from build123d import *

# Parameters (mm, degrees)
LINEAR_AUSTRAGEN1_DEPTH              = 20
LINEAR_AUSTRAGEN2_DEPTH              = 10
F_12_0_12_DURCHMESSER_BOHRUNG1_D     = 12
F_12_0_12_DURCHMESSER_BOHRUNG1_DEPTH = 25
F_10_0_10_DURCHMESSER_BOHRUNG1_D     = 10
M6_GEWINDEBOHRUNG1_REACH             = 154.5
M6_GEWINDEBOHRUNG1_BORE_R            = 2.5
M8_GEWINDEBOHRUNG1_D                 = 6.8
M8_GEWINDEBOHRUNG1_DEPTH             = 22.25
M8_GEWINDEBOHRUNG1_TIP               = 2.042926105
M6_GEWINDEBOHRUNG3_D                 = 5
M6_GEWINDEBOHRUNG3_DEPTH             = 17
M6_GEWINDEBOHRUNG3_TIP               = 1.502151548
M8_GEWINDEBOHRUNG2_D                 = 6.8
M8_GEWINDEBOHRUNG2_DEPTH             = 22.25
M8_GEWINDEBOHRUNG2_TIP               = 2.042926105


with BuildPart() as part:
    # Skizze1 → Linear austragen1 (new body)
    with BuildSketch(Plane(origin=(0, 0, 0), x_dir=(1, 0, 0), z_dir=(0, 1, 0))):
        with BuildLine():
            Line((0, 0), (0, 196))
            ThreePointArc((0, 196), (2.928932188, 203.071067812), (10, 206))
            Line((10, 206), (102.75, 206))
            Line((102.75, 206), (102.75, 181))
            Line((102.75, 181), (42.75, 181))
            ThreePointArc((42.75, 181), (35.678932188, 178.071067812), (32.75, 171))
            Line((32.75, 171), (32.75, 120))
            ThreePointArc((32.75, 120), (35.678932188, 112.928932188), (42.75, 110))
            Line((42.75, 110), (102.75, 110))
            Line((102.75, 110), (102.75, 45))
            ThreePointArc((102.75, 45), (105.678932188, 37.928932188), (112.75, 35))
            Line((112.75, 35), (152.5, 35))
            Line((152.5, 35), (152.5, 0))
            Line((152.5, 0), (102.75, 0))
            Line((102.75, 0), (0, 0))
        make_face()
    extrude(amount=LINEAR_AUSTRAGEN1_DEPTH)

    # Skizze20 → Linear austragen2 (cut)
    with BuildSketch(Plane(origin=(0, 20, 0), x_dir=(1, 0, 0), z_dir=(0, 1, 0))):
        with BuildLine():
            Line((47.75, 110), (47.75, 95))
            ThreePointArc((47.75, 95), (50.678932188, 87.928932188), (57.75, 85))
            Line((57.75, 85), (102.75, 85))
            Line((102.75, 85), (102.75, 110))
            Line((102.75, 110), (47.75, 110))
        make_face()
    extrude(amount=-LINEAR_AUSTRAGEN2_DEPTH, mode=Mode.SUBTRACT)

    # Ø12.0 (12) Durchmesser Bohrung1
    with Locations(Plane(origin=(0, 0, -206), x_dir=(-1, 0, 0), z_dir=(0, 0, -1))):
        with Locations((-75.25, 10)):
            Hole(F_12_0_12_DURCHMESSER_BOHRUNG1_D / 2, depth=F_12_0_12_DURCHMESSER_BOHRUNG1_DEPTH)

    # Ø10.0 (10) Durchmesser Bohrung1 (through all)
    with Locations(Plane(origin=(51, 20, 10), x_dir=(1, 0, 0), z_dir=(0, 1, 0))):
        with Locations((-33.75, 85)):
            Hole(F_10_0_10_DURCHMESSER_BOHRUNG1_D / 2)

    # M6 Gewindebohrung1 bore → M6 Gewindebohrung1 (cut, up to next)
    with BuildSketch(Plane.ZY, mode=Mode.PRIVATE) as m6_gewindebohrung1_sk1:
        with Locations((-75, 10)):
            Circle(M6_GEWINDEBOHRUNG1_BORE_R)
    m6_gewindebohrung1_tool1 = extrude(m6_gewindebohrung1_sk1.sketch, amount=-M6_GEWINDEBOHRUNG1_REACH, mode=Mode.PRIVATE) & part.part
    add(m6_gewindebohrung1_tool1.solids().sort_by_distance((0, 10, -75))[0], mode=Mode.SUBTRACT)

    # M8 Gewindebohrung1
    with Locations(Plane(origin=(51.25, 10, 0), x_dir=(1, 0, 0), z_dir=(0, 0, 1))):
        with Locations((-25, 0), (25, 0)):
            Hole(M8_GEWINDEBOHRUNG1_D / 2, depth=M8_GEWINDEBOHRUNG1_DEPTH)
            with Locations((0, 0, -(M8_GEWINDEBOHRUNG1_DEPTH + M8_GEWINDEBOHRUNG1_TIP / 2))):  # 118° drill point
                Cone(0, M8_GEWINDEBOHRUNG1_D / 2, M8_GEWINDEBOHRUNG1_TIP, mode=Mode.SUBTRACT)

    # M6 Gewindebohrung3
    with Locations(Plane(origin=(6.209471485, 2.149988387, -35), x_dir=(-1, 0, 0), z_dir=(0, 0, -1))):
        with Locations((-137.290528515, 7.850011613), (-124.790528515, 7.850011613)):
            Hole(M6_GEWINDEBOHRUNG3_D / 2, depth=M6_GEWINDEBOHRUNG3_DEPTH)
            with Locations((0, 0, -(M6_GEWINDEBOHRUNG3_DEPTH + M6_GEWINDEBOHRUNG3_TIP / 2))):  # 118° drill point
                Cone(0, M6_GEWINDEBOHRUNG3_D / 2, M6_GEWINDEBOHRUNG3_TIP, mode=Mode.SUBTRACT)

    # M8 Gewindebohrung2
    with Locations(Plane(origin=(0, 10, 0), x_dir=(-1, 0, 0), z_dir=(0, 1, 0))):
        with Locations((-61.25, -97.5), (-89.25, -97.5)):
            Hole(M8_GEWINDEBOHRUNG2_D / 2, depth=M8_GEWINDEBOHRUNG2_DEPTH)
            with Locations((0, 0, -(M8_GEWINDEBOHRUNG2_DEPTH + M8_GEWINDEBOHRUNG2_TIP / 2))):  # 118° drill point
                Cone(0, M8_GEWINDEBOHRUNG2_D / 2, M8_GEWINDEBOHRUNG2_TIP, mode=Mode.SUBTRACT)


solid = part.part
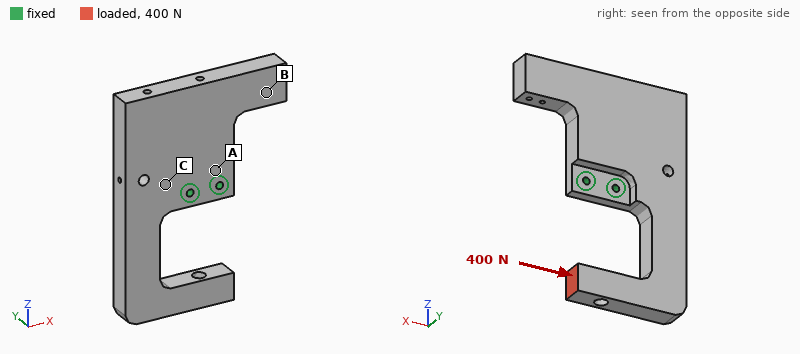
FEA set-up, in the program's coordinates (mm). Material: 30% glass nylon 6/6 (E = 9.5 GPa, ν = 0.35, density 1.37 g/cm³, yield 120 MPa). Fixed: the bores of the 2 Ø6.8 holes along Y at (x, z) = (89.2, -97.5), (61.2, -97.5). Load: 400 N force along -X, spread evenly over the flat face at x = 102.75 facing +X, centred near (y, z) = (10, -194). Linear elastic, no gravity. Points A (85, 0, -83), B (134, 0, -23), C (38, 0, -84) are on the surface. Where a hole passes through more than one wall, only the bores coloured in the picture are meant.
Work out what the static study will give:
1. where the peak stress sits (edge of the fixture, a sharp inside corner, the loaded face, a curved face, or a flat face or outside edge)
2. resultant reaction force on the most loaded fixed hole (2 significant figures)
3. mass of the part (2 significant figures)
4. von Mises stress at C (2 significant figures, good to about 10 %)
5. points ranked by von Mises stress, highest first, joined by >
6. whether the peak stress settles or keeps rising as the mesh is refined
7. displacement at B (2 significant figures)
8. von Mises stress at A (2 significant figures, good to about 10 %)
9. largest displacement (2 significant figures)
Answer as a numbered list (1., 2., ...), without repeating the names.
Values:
1. edge of the fixture
2. 1.3 kN
3. 460 g
4. 3.0 MPa
5. A > C > B
6. keeps rising
7. 0.11 mm
8. 4.6 MPa
9. 0.57 mm
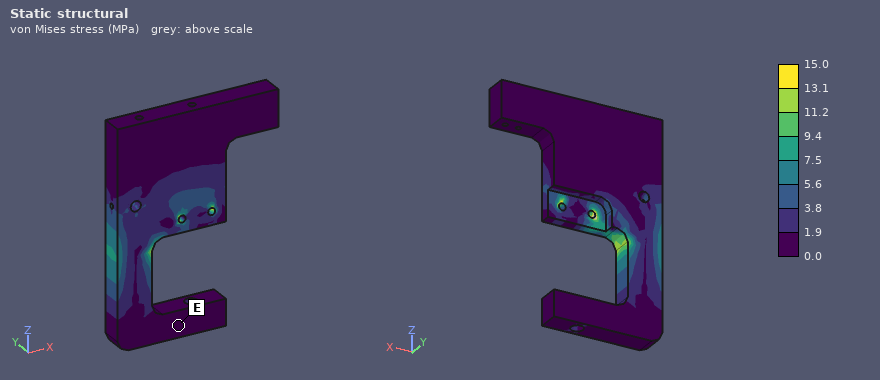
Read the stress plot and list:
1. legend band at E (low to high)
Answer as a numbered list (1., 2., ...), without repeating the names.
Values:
1. 0.0 to 1.9 MPa
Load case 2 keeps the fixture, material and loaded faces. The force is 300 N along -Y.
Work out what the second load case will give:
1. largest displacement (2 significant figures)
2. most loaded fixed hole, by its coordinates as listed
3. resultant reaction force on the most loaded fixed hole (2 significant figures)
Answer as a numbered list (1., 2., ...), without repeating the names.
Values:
1. 3.1 mm
2. (89.2, -97.5)
3. 360 N
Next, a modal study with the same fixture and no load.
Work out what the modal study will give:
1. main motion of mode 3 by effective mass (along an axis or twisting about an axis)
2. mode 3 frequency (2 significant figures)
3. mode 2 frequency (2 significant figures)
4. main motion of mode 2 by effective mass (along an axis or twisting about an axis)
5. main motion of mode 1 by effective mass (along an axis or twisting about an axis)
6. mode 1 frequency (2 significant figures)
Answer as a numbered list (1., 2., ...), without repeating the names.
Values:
1. along Y
2. 470 Hz
3. 430 Hz
4. along Y
5. twisting about X
6. 210 Hz
